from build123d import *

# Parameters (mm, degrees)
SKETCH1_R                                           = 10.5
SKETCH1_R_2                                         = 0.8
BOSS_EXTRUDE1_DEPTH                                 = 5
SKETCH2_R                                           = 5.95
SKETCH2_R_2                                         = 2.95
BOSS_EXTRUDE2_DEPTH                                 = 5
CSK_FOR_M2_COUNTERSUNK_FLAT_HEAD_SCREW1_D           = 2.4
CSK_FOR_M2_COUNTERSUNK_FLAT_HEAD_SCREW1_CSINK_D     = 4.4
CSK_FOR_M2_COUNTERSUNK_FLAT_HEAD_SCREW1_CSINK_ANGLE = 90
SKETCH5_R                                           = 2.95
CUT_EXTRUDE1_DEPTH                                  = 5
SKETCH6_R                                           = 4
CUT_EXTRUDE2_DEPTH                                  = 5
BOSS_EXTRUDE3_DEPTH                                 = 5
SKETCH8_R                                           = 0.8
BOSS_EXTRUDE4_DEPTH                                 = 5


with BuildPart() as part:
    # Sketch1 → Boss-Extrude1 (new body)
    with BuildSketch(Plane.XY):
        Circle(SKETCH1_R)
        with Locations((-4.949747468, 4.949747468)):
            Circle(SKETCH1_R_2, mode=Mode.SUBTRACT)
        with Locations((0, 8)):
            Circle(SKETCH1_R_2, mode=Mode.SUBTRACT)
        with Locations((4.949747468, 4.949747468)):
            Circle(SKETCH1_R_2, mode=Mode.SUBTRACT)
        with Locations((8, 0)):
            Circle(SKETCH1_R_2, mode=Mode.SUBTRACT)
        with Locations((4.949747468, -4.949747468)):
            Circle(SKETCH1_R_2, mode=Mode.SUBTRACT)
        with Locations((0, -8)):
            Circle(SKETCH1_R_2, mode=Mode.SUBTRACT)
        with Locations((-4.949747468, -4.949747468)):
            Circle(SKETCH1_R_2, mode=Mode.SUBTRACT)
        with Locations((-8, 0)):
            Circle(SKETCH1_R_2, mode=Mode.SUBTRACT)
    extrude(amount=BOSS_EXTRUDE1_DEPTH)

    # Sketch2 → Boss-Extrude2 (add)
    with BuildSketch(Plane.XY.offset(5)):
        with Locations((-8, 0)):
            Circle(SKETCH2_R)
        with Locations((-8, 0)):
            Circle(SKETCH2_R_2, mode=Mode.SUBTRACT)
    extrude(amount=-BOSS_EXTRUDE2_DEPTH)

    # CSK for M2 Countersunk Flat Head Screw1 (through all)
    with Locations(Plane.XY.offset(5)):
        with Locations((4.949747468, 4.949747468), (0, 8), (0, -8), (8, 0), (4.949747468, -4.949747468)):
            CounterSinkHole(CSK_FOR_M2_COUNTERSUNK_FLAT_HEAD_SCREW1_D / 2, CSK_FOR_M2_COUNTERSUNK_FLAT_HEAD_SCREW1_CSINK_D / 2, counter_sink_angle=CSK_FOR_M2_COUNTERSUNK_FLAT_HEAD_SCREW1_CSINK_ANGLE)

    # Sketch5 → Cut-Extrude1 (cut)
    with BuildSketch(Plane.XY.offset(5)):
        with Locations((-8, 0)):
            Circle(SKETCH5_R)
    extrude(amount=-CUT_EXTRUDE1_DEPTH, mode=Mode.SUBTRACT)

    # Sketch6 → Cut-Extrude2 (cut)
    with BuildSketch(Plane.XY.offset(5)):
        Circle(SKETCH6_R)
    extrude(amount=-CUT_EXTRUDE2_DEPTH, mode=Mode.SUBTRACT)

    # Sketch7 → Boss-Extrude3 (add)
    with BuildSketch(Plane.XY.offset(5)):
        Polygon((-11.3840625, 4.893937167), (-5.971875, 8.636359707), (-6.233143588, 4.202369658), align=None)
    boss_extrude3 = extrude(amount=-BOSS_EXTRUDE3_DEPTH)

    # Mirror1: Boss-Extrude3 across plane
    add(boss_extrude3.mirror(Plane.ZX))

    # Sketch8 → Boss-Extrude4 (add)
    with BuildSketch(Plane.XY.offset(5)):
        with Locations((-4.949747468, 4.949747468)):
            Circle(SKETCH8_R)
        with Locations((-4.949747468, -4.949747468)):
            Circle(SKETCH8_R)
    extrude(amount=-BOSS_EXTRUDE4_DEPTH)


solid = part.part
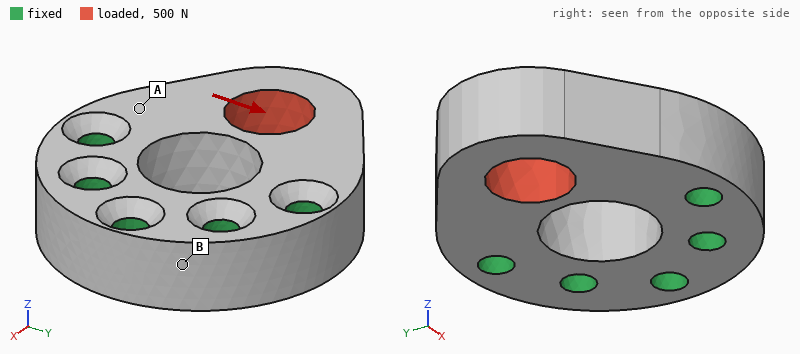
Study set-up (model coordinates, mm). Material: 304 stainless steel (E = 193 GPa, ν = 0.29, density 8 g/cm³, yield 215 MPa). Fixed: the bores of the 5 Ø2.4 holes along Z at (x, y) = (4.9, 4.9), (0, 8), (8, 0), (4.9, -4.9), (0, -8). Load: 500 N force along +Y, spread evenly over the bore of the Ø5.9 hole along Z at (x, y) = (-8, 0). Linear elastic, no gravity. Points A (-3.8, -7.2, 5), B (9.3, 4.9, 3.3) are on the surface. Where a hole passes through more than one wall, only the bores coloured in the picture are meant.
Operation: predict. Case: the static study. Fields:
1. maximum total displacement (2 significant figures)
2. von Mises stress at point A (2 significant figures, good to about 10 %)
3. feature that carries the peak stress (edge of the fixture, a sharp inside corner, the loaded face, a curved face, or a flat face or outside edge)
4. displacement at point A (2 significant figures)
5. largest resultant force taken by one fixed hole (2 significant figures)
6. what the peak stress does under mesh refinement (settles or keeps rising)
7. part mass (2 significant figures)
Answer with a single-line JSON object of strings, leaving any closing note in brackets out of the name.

{"maximum total displacement": "2.5 µm", "von Mises stress at point A": "11 MPa", "feature that carries the peak stress": "edge of the fixture", "displacement at point A": "0.70 µm", "largest resultant force taken by one fixed hole": "350 N", "what the peak stress does under mesh refinement": "keeps rising", "part mass": "11 g"}
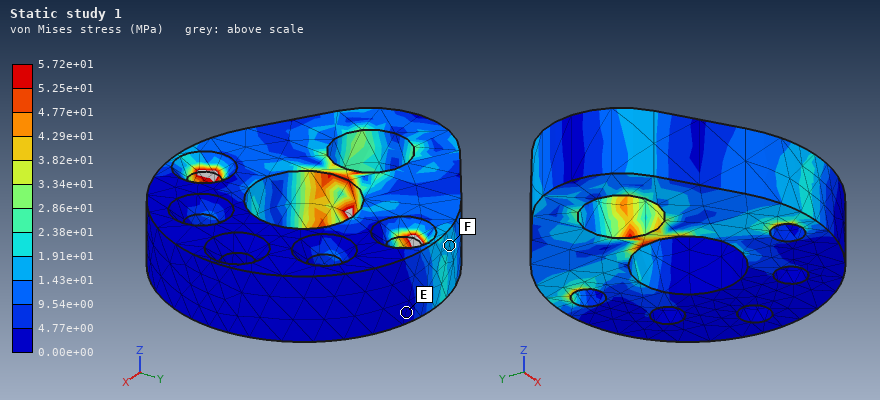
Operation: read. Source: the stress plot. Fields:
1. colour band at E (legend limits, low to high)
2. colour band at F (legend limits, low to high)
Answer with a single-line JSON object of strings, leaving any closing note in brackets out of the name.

{"colour band at E": "0.00e+00 to 4.77e+00 MPa", "colour band at F": "1.43e+01 to 1.91e+01 MPa"}
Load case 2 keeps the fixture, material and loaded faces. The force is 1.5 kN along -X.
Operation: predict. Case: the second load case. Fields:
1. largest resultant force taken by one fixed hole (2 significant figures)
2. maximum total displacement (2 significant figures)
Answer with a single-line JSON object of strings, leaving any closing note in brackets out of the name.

{"largest resultant force taken by one fixed hole": "660 N", "maximum total displacement": "2.8 µm"}
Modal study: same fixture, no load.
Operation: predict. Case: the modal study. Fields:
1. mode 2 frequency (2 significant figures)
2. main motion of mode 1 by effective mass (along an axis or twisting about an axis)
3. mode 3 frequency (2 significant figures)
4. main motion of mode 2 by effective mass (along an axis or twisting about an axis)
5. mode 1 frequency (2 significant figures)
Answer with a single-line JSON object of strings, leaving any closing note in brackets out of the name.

{"mode 2 frequency": "41 kHz", "main motion of mode 1 by effective mass": "along Z", "mode 3 frequency": "48 kHz", "main motion of mode 2 by effective mass": "along Y", "mode 1 frequency": "21 kHz"}
